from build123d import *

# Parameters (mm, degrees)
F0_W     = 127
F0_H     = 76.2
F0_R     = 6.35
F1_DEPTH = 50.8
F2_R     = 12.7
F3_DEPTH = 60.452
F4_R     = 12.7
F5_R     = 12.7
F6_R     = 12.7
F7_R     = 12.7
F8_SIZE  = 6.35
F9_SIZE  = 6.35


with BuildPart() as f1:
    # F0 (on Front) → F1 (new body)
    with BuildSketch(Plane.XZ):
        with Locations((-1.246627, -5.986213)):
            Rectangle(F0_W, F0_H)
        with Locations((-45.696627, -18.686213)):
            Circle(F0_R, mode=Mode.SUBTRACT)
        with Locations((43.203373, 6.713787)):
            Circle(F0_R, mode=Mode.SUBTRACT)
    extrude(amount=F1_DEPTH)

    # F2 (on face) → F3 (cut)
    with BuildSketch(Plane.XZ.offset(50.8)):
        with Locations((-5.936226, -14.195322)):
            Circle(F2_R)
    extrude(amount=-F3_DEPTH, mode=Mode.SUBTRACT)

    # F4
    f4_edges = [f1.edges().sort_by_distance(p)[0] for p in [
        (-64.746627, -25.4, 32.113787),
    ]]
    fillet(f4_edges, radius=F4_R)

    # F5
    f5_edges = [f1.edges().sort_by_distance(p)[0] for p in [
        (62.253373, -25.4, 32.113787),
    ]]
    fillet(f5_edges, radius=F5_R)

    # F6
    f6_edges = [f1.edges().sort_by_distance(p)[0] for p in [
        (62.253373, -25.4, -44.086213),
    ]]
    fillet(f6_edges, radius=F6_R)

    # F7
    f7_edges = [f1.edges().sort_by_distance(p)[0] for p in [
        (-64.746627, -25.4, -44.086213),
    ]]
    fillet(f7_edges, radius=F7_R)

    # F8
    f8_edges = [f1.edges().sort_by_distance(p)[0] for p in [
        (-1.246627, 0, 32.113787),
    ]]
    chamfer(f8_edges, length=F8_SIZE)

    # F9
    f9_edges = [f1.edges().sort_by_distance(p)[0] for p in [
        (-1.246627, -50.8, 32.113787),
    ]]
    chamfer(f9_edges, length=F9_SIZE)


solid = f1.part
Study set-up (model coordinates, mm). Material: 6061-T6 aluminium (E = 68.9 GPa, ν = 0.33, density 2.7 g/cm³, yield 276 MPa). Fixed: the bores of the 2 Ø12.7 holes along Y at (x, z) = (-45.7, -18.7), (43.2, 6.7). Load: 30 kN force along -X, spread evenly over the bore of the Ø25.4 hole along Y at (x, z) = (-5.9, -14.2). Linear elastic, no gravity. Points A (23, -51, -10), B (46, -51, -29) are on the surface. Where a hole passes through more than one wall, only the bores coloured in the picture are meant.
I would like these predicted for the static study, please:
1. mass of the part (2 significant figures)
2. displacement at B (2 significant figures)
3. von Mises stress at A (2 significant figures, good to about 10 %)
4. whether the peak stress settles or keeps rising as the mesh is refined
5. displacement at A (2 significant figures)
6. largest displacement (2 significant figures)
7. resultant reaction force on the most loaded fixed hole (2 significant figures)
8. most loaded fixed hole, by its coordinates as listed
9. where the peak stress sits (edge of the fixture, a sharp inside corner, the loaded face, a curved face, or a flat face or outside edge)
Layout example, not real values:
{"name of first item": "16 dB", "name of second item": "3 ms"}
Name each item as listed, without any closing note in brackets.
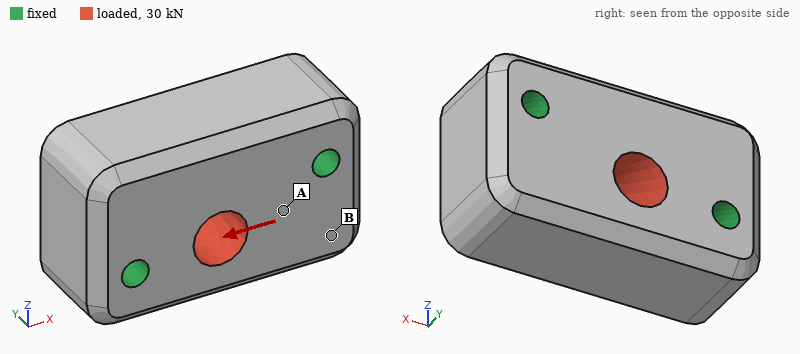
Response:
{"mass of the part": "1.2 kg", "displacement at B": "4.7 µm", "von Mises stress at A": "7.4 MPa", "whether the peak stress settles or keeps rising as the mesh is refined": "keeps rising", "displacement at A": "3.9 µm", "largest displacement": "7.0 µm", "resultant reaction force on the most loaded fixed hole": "17 kN", "most loaded fixed hole, by its coordinates as listed": "(-45.7, -18.7)", "where the peak stress sits": "edge of the fixture"}
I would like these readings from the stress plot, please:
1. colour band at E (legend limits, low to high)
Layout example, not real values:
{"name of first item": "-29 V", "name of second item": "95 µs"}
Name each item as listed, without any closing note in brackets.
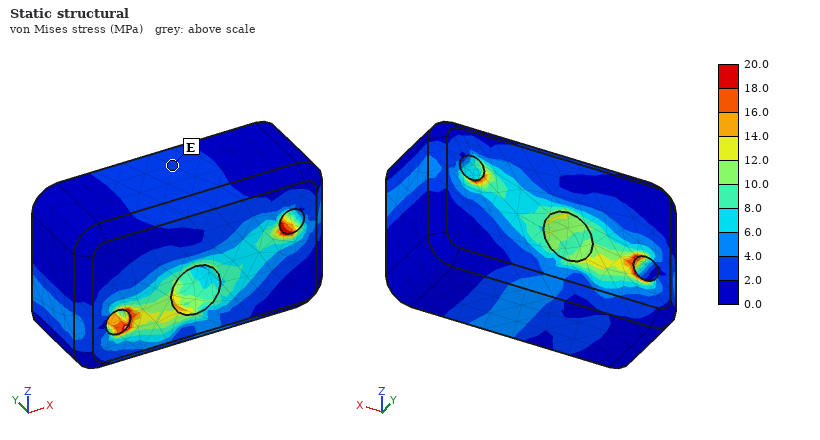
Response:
{"colour band at E": "2.0 to 4.0 MPa"}
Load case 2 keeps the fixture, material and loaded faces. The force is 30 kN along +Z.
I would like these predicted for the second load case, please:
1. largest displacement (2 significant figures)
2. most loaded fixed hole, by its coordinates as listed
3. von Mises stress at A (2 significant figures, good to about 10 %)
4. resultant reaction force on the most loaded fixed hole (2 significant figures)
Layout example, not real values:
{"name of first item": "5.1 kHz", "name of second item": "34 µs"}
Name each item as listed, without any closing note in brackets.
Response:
{"largest displacement": "12 µm", "most loaded fixed hole, by its coordinates as listed": "(-45.7, -18.7)", "von Mises stress at A": "8.5 MPa", "resultant reaction force on the most loaded fixed hole": "17 kN"}
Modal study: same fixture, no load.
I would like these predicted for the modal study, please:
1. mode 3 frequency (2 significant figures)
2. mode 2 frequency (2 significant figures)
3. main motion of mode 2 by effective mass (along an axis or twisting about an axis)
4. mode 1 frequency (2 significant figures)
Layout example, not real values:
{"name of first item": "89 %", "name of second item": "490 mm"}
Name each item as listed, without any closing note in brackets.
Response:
{"mode 3 frequency": "12 kHz", "mode 2 frequency": "11 kHz", "main motion of mode 2 by effective mass": "along Y", "mode 1 frequency": "9800 Hz"}
